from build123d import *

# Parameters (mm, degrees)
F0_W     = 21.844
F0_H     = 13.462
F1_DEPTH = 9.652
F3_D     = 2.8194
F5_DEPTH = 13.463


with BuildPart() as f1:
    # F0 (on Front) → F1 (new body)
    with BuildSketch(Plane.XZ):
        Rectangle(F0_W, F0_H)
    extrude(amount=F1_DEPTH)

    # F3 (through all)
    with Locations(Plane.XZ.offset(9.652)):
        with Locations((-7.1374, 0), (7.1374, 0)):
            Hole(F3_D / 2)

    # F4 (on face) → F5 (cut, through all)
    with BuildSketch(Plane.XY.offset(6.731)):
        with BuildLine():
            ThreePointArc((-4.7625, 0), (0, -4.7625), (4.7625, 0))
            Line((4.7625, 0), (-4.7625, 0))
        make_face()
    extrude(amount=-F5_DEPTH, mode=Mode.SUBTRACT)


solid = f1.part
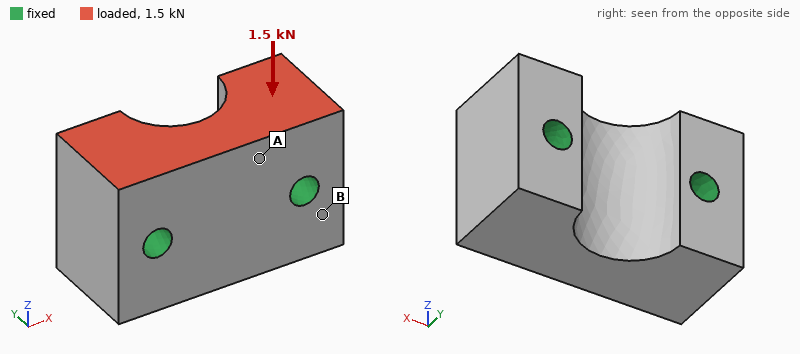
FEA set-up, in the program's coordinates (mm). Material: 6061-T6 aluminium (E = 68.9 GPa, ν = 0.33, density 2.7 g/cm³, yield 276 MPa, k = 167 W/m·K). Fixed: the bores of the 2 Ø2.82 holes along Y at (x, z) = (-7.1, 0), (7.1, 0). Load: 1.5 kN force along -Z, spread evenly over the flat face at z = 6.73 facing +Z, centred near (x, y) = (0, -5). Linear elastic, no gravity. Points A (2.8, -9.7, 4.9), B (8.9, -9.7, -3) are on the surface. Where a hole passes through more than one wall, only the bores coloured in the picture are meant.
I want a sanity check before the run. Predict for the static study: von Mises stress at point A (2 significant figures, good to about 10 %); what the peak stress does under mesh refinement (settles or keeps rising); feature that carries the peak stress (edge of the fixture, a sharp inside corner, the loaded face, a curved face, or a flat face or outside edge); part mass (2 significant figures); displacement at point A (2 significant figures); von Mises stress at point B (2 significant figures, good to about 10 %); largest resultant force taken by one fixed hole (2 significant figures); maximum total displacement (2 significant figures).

8.0 MPa
keeps rising
edge of the fixture
6.0 g
1.1 µm
2.6 MPa
750 N
1.5 µm
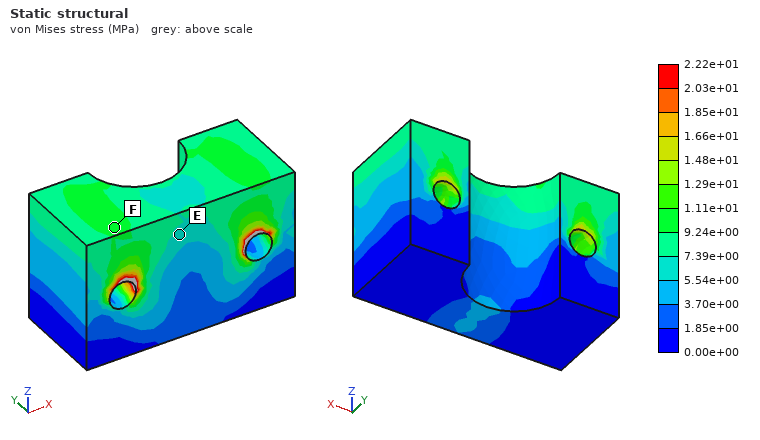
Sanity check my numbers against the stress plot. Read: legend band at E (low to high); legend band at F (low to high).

5.54e+00 to 7.39e+00 MPa
9.24e+00 to 1.11e+01 MPa
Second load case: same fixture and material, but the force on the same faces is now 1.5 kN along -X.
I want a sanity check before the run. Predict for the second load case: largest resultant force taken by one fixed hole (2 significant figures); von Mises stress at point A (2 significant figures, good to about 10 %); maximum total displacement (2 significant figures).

890 N
20 MPa
5.5 µm
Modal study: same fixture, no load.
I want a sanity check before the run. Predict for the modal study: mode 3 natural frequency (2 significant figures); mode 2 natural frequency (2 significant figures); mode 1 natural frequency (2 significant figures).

85 kHz
84 kHz
76 kHz
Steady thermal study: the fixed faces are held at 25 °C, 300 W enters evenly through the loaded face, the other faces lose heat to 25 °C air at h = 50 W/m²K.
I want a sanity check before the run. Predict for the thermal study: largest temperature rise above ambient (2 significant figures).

74 K
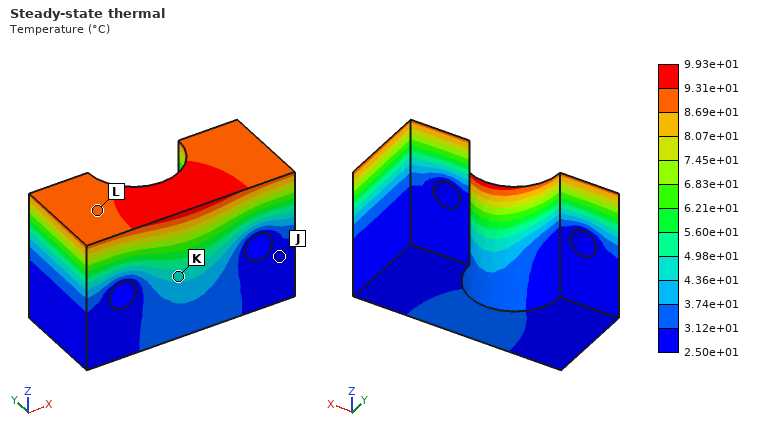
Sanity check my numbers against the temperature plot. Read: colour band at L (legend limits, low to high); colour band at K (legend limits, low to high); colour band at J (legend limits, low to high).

8.69e+01 to 9.31e+01 °C
4.36e+01 to 4.98e+01 °C
2.50e+01 to 3.12e+01 °C
